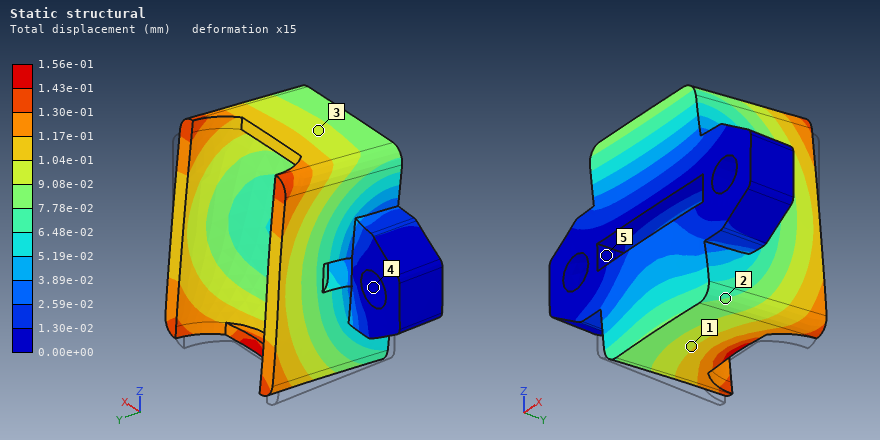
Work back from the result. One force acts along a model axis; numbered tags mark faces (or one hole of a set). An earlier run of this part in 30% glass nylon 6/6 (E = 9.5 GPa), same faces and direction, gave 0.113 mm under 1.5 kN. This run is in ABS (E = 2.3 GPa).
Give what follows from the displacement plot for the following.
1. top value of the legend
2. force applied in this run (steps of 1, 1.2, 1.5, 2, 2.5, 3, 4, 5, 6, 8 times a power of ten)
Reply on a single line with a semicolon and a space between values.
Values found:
1.56e-01 mm; 500 N
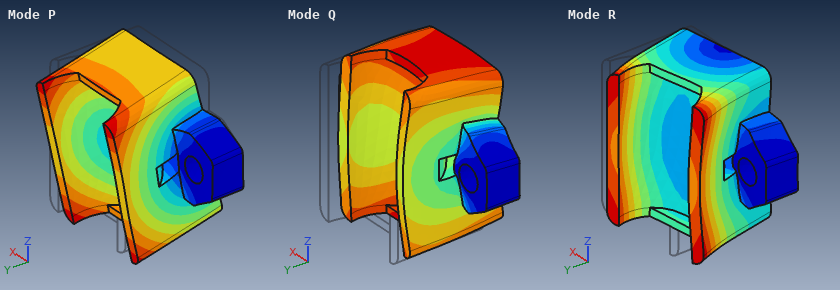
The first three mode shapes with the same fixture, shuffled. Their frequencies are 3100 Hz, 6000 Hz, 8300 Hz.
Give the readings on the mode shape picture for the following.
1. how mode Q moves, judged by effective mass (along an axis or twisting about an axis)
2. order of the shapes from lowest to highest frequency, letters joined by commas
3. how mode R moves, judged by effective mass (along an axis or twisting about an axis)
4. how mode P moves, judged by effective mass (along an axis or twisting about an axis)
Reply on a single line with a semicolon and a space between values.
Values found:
along Y; P, Q, R; along X; along Z
